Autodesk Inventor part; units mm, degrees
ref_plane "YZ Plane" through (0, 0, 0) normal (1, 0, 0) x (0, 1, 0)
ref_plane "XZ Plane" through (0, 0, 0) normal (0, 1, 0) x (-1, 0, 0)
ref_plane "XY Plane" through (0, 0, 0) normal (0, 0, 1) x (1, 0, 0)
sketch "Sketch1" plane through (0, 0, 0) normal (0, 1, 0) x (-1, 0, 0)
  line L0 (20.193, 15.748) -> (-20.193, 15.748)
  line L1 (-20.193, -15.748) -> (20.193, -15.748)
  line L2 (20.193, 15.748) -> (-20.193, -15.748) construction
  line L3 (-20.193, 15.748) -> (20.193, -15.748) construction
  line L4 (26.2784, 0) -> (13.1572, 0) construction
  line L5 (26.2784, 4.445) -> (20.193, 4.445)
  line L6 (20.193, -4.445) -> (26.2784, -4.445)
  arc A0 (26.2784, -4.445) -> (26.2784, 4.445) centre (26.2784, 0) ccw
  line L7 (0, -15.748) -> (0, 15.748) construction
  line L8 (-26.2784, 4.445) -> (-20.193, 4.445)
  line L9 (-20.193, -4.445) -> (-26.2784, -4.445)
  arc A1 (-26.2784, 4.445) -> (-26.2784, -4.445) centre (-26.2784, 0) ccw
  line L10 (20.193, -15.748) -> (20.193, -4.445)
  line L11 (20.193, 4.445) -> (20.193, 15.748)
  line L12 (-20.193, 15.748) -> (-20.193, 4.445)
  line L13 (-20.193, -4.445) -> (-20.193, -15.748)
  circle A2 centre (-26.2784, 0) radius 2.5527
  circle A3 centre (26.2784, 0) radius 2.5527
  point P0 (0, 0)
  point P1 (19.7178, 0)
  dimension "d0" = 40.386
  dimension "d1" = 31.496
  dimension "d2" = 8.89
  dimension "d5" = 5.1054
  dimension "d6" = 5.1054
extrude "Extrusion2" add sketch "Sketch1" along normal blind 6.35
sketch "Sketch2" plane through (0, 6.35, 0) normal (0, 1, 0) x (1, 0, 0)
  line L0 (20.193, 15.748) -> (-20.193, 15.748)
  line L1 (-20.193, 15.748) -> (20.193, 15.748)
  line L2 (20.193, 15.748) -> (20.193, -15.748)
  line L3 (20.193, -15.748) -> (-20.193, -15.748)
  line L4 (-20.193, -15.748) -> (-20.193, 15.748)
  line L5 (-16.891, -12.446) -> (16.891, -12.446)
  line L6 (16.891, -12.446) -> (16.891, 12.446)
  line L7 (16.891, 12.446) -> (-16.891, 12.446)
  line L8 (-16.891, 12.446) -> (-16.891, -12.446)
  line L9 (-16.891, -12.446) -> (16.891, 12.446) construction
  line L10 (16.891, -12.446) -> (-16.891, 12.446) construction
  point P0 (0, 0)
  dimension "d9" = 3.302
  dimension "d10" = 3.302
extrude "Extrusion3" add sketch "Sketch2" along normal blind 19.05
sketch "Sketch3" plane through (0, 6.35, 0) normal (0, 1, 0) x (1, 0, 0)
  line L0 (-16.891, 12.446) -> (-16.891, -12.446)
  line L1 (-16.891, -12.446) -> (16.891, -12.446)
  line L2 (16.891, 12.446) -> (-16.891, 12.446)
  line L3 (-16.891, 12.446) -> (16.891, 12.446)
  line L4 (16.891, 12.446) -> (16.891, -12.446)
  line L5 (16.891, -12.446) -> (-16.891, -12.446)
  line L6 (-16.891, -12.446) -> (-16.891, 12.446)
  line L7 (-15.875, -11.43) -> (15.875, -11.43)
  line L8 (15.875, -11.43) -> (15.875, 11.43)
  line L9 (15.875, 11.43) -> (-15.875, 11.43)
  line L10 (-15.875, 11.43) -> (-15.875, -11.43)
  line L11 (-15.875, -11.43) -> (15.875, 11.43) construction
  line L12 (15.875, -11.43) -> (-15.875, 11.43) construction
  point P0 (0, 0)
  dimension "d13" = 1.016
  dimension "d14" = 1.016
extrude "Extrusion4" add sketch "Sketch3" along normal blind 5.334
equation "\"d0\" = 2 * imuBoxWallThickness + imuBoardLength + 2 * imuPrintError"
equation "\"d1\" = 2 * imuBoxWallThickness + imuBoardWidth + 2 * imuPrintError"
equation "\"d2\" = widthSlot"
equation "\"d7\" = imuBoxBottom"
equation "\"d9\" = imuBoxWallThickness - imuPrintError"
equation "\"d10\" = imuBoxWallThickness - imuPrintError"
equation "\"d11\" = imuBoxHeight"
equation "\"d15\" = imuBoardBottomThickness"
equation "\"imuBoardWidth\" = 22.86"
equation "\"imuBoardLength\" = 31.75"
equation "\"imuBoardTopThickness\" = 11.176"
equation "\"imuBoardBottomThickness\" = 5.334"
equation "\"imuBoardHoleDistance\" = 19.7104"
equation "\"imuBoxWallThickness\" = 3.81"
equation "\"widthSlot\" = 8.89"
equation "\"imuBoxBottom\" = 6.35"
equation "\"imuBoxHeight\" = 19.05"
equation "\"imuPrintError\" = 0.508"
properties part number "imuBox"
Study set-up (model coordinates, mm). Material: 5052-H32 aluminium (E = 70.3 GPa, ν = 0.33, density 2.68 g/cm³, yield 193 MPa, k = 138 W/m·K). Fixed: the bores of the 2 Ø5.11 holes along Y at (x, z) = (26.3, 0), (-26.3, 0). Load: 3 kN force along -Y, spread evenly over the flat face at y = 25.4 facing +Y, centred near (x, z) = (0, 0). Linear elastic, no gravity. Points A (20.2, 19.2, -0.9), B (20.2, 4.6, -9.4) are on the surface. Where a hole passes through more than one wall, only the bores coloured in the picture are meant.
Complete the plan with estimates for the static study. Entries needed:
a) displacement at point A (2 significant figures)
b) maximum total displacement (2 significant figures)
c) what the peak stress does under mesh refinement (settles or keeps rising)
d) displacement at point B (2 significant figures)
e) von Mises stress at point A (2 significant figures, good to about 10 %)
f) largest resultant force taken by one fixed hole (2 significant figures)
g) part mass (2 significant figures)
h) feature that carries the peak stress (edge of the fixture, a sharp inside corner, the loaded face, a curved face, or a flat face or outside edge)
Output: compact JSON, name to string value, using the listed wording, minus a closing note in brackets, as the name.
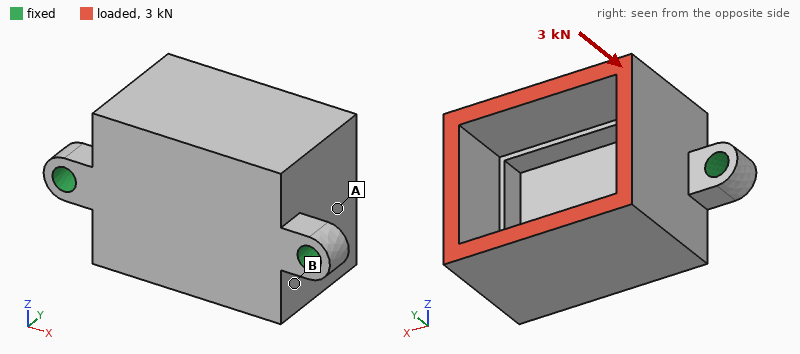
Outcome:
{"displacement at point A": "14 µm", "maximum total displacement": "22 µm", "what the peak stress does under mesh refinement": "keeps rising", "displacement at point B": "13 µm", "von Mises stress at point A": "11 MPa", "largest resultant force taken by one fixed hole": "1.5 kN", "part mass": "48 g", "feature that carries the peak stress": "edge of the fixture"}
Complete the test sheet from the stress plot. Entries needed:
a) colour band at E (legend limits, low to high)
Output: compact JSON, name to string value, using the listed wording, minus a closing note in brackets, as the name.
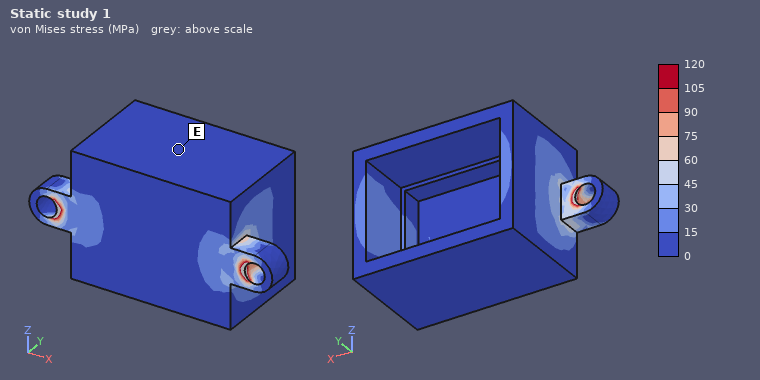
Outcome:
{"colour band at E": "0 to 15 MPa"}
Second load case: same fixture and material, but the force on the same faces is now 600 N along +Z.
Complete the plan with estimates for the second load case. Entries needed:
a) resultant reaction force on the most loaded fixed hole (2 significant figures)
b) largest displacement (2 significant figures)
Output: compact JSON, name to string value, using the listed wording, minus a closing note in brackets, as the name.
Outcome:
{"resultant reaction force on the most loaded fixed hole": "300 N", "largest displacement": "0.11 mm"}
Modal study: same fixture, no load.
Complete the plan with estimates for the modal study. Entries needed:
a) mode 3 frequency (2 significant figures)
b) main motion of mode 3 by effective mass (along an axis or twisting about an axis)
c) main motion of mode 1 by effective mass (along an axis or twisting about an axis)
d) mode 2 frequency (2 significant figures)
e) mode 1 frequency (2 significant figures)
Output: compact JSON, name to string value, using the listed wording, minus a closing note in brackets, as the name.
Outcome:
{"mode 3 frequency": "9800 Hz", "main motion of mode 3 by effective mass": "along Y", "main motion of mode 1 by effective mass": "along Z", "mode 2 frequency": "8300 Hz", "mode 1 frequency": "3300 Hz"}
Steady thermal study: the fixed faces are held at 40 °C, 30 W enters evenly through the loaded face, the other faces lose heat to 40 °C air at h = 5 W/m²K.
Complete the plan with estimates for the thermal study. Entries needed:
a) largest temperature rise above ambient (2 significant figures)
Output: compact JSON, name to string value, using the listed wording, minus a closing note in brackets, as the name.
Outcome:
{"largest temperature rise above ambient": "24 K"}
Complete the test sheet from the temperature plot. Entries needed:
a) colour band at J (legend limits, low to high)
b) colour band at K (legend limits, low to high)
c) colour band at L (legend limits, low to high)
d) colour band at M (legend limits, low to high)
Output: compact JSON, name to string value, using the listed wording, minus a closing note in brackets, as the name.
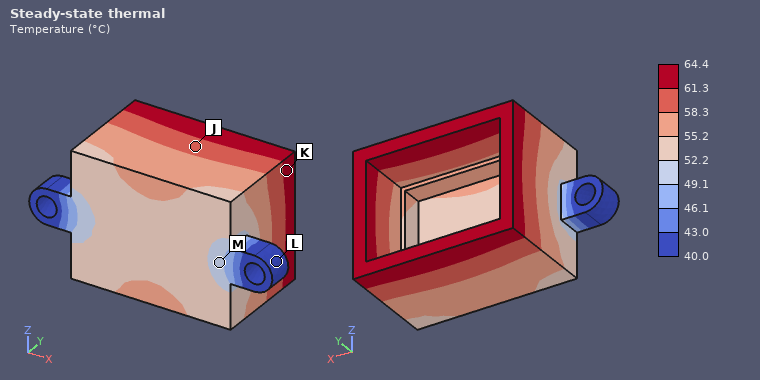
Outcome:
{"colour band at J": "58.3 to 61.3 °C", "colour band at K": "61.3 to 64.4 °C", "colour band at L": "40.0 to 43.0 °C", "colour band at M": "49.1 to 52.2 °C"}
